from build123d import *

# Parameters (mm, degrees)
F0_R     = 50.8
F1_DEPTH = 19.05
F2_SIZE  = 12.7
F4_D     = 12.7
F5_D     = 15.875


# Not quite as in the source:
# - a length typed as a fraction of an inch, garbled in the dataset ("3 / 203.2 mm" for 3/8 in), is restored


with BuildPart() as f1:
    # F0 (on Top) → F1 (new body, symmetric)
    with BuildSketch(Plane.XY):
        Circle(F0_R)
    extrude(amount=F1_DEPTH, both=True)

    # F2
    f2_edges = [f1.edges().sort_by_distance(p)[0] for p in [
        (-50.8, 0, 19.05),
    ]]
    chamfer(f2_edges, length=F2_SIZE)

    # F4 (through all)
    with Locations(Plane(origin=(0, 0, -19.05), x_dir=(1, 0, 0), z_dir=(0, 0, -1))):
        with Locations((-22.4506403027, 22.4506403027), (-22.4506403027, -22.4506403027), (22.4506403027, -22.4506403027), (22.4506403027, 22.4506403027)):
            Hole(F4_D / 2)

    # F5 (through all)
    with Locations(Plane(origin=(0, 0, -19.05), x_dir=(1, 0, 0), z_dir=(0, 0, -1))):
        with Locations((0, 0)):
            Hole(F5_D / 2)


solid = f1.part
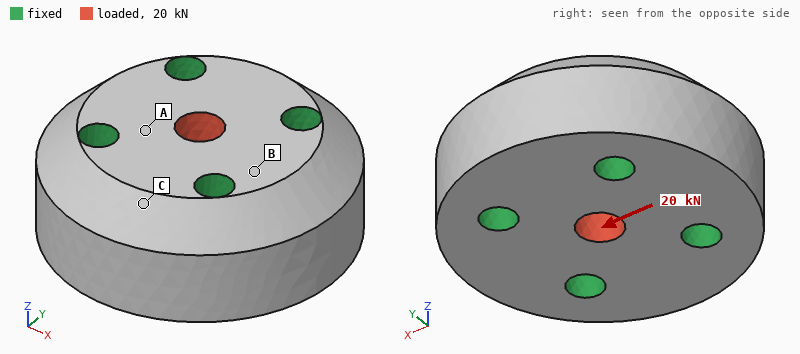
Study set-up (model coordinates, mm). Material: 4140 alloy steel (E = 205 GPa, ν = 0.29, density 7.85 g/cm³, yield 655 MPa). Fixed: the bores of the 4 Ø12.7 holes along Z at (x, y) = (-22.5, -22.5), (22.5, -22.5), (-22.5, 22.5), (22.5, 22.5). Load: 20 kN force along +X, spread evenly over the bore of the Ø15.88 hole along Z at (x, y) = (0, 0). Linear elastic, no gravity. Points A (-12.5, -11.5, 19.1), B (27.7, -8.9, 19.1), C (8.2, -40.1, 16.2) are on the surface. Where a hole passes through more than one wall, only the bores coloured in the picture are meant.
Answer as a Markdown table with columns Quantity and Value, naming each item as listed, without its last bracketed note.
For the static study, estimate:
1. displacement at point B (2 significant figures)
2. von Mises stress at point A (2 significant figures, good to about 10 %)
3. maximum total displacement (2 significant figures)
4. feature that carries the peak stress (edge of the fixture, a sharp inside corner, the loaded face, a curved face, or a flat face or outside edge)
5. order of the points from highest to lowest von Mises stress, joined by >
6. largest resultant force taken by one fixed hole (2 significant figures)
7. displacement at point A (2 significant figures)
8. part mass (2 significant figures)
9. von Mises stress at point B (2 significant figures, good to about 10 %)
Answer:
| Quantity | Value |
|---|---|
| displacement at point B | 0.36 µm |
| von Mises stress at point A | 7.9 MPa |
| maximum total displacement | 1.1 µm |
| feature that carries the peak stress | the loaded face |
| order of the points from highest to lowest von Mises stress, joined by > | A > B > C |
| largest resultant force taken by one fixed hole | 5.3 kN |
| displacement at point A | 0.43 µm |
| part mass | 2.0 kg |
| von Mises stress at point B | 3.8 MPa |
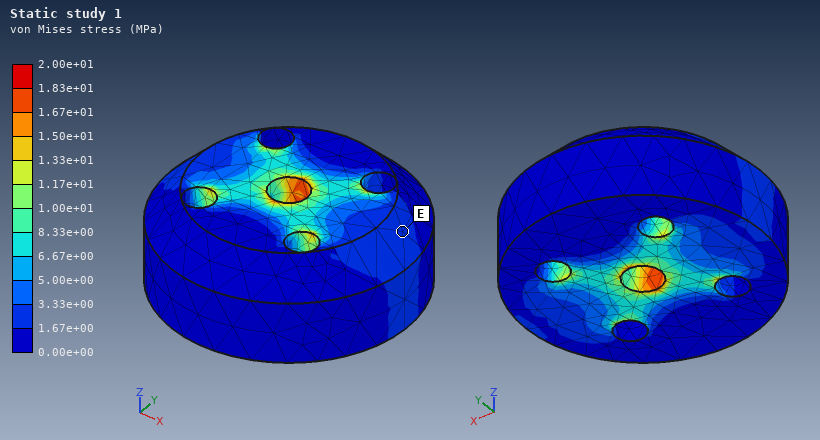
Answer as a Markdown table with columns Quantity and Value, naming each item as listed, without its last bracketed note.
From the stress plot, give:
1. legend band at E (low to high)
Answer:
| Quantity | Value |
|---|---|
| legend band at E | 1.67e+00 to 3.33e+00 MPa |
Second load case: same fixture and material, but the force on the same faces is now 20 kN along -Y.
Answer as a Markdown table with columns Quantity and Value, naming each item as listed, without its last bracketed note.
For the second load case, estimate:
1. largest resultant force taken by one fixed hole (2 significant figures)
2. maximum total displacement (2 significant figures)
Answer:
| Quantity | Value |
|---|---|
| largest resultant force taken by one fixed hole | 5.3 kN |
| maximum total displacement | 1.1 µm |
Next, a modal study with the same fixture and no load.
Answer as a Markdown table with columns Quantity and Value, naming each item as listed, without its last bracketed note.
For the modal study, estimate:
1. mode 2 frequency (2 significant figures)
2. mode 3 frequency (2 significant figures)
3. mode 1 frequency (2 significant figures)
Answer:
| Quantity | Value |
|---|---|
| mode 2 frequency | 26 kHz |
| mode 3 frequency | 26 kHz |
| mode 1 frequency | 25 kHz |
